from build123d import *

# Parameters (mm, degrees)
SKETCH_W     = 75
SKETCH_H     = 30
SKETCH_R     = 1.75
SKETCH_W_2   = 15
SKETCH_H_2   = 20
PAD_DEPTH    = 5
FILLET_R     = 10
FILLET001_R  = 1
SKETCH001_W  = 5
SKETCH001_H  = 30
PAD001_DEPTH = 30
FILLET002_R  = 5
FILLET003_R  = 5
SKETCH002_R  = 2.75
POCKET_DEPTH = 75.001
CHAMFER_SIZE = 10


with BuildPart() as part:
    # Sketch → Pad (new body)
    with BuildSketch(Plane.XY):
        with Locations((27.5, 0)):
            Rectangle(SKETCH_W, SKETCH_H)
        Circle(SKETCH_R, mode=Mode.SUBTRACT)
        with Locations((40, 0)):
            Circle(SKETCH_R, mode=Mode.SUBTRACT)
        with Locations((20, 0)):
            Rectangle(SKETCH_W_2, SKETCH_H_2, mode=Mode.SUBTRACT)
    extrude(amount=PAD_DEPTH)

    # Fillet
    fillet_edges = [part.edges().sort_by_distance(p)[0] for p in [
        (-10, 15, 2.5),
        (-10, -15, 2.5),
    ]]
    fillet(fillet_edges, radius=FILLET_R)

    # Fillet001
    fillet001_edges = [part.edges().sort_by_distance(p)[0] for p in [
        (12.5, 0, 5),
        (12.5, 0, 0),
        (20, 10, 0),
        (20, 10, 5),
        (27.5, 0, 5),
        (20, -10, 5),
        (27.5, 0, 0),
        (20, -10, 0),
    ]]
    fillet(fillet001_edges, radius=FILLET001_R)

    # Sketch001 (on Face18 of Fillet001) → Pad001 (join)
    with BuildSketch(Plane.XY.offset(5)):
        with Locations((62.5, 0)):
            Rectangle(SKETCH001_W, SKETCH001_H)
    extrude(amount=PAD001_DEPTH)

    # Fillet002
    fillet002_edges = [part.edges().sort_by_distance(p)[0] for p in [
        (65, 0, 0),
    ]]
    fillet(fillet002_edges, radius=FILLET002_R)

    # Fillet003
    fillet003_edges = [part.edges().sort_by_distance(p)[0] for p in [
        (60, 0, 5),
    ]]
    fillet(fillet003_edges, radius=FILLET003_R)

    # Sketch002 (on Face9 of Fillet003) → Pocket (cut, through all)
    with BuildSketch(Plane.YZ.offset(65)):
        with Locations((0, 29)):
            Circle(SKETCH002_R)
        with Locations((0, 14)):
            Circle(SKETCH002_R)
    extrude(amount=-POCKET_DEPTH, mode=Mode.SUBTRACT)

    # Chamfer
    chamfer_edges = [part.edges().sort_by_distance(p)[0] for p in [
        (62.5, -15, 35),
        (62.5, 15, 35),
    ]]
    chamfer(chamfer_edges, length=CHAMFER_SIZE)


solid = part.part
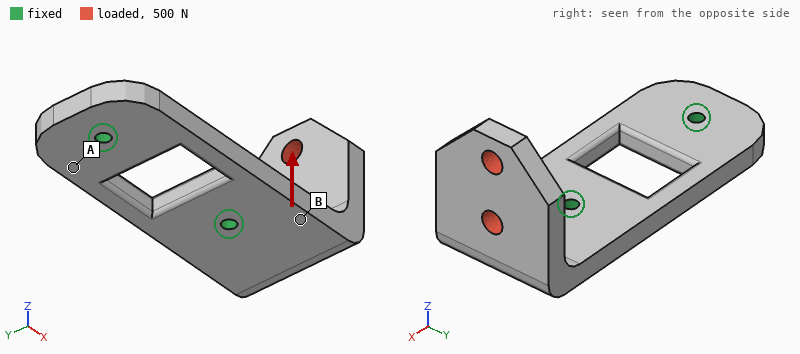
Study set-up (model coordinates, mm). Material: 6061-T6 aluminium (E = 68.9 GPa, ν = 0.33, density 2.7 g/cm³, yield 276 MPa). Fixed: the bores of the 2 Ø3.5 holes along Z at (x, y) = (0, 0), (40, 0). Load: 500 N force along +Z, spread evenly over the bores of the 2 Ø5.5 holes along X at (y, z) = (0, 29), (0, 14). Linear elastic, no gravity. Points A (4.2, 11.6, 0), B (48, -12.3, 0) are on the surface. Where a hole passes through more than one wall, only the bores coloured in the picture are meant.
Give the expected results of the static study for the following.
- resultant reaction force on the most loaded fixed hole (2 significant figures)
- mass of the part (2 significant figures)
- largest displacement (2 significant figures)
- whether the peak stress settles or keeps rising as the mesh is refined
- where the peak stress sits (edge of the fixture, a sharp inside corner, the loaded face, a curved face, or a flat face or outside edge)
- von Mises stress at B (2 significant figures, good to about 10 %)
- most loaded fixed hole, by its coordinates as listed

570 N
36 g
0.25 mm
keeps rising
edge of the fixture
49 MPa
(40, 0)
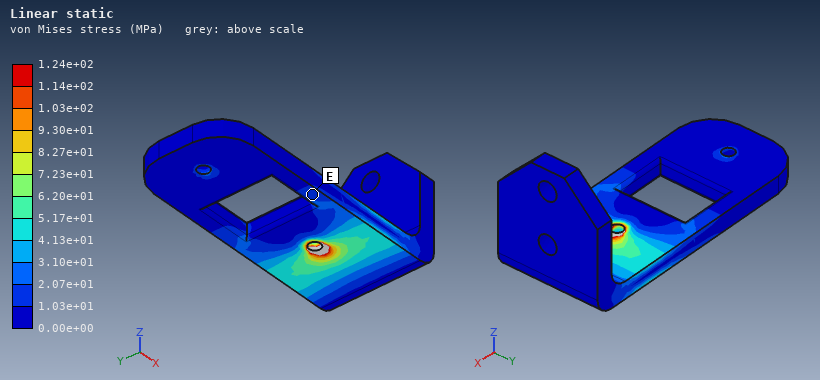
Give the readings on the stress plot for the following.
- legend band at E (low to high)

1.03e+01 to 2.07e+01 MPa
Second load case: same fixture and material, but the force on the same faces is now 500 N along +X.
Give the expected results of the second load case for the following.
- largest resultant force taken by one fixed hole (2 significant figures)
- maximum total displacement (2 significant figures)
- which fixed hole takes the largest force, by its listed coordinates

450 N
0.42 mm
(40, 0)
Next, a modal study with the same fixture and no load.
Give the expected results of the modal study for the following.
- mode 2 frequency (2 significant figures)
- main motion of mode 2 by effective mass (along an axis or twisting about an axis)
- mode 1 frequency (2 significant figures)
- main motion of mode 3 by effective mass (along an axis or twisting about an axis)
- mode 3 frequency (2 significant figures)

2800 Hz
along Y
2000 Hz
along Z
5900 Hz
